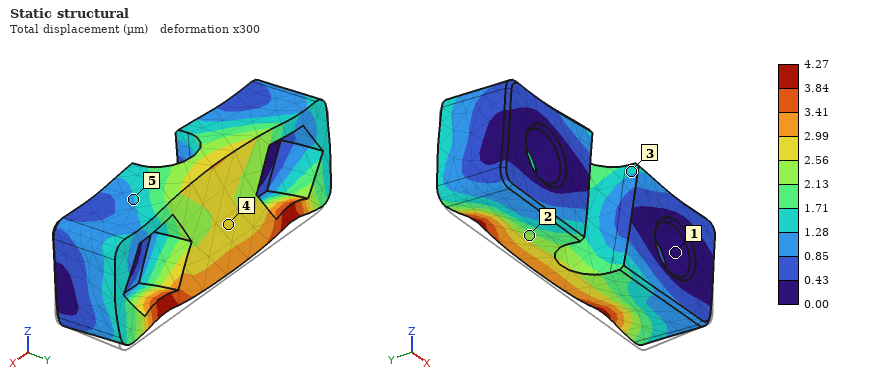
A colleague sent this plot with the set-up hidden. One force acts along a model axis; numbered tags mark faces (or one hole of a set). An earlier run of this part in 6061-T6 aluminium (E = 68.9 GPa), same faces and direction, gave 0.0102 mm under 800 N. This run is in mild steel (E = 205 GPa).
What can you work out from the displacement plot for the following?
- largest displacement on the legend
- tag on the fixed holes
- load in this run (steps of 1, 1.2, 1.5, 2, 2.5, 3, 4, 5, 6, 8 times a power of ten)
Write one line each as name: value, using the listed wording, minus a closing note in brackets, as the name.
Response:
largest displacement on the legend: 4.27 µm
tag on the fixed holes: 1
load in this run: 1 kN
